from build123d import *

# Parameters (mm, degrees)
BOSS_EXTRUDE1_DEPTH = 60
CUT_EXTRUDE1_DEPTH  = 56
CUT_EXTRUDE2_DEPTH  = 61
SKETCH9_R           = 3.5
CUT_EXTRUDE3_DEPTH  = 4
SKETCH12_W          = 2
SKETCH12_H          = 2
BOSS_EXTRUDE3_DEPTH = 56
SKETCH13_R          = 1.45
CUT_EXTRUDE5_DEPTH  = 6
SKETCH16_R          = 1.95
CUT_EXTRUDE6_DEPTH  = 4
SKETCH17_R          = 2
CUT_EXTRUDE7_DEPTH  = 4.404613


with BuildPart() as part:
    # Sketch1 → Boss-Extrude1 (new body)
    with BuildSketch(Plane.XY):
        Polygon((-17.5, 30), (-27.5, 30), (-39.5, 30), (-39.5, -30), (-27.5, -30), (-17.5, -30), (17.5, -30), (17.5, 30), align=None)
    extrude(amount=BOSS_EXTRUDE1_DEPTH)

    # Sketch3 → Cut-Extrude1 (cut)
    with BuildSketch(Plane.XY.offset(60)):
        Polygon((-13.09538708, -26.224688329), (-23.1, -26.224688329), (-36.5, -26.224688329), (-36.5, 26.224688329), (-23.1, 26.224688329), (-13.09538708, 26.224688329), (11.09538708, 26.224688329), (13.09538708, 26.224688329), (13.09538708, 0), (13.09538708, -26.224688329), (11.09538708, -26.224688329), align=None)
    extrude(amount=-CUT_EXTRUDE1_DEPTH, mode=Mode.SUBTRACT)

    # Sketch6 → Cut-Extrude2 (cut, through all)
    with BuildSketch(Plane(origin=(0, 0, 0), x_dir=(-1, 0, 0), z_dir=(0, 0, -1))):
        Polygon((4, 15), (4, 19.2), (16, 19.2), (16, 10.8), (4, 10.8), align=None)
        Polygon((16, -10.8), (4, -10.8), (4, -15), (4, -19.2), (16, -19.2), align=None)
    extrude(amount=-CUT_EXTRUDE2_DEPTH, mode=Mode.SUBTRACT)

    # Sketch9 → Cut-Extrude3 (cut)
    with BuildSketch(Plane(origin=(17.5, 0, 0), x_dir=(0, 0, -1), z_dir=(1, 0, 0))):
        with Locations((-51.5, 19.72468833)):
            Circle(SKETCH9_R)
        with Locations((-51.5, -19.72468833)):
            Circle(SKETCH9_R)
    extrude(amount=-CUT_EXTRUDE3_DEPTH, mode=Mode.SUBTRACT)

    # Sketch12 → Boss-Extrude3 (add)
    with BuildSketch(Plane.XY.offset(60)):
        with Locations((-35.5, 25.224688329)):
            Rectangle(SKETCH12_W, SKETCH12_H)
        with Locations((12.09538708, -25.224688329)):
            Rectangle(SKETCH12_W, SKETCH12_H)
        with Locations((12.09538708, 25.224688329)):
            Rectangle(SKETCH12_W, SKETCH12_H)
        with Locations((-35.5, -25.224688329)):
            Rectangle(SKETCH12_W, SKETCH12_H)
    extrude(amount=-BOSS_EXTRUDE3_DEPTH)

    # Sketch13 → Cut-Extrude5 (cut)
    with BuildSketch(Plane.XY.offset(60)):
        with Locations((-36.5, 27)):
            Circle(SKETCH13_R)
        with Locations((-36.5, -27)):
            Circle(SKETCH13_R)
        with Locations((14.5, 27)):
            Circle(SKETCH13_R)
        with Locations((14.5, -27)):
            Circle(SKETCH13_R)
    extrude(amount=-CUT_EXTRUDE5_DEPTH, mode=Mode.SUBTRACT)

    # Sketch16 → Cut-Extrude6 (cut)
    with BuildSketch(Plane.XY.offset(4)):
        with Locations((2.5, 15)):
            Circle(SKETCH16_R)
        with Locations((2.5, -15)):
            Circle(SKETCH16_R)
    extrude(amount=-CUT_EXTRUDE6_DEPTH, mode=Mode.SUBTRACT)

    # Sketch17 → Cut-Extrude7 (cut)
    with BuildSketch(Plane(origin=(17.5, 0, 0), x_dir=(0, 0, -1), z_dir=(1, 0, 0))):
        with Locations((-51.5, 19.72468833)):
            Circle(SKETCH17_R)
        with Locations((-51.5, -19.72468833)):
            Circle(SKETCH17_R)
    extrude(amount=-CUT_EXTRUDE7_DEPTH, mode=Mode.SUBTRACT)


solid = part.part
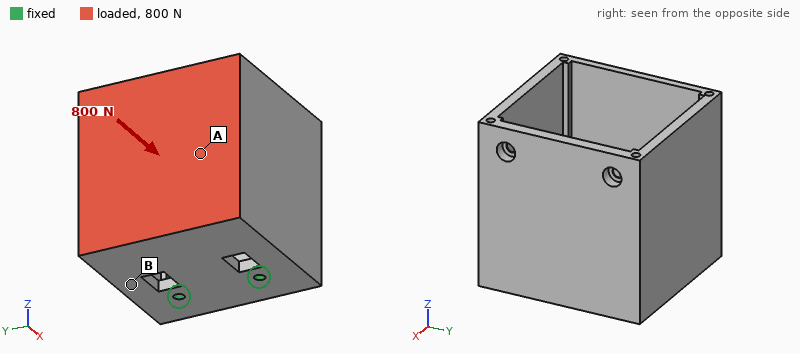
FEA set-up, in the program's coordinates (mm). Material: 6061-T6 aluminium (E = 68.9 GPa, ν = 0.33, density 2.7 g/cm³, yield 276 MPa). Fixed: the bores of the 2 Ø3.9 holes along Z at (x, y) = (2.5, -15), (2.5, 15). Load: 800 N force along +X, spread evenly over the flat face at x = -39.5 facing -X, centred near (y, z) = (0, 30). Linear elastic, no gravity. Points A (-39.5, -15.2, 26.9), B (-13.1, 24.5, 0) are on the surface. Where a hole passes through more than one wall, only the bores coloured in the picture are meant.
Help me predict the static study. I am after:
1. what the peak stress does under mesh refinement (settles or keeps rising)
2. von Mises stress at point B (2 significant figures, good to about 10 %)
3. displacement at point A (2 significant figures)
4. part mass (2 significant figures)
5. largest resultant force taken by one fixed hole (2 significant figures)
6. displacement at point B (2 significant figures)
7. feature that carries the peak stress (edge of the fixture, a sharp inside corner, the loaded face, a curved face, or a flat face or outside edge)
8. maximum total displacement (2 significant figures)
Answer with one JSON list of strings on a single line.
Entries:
["keeps rising", "25 MPa", "0.31 mm", "160 g", "420 N", "0.100 mm", "edge of the fixture", "0.48 mm"]
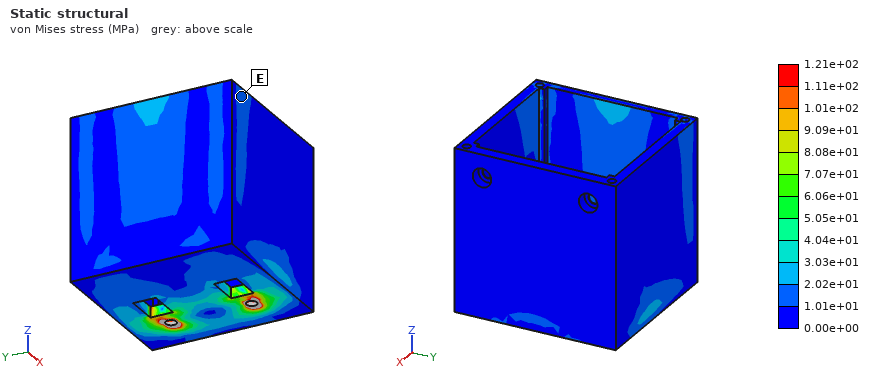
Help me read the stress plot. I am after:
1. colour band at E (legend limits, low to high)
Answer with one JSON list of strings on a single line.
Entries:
["1.01e+01 to 2.02e+01 MPa"]
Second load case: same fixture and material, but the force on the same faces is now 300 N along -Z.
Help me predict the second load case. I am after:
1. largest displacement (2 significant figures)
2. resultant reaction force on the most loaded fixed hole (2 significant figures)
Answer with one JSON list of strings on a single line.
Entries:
["0.26 mm", "160 N"]
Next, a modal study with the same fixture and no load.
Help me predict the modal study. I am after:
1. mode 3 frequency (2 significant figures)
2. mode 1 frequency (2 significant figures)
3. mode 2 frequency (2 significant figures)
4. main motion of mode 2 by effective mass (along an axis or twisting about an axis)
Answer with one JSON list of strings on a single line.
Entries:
["2300 Hz", "630 Hz", "1600 Hz", "along Y"]
